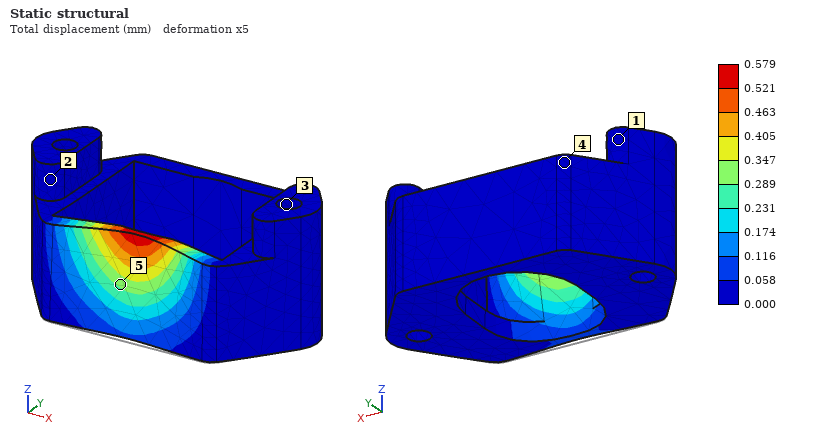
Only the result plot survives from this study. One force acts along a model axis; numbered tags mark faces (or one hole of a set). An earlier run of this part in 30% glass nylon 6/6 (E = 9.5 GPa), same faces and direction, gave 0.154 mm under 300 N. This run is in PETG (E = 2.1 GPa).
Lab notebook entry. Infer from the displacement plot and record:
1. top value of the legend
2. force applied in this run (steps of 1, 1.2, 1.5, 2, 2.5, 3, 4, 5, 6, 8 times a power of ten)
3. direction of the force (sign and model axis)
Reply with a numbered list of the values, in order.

1. 0.579 mm
2. 250 N
3. +Y
